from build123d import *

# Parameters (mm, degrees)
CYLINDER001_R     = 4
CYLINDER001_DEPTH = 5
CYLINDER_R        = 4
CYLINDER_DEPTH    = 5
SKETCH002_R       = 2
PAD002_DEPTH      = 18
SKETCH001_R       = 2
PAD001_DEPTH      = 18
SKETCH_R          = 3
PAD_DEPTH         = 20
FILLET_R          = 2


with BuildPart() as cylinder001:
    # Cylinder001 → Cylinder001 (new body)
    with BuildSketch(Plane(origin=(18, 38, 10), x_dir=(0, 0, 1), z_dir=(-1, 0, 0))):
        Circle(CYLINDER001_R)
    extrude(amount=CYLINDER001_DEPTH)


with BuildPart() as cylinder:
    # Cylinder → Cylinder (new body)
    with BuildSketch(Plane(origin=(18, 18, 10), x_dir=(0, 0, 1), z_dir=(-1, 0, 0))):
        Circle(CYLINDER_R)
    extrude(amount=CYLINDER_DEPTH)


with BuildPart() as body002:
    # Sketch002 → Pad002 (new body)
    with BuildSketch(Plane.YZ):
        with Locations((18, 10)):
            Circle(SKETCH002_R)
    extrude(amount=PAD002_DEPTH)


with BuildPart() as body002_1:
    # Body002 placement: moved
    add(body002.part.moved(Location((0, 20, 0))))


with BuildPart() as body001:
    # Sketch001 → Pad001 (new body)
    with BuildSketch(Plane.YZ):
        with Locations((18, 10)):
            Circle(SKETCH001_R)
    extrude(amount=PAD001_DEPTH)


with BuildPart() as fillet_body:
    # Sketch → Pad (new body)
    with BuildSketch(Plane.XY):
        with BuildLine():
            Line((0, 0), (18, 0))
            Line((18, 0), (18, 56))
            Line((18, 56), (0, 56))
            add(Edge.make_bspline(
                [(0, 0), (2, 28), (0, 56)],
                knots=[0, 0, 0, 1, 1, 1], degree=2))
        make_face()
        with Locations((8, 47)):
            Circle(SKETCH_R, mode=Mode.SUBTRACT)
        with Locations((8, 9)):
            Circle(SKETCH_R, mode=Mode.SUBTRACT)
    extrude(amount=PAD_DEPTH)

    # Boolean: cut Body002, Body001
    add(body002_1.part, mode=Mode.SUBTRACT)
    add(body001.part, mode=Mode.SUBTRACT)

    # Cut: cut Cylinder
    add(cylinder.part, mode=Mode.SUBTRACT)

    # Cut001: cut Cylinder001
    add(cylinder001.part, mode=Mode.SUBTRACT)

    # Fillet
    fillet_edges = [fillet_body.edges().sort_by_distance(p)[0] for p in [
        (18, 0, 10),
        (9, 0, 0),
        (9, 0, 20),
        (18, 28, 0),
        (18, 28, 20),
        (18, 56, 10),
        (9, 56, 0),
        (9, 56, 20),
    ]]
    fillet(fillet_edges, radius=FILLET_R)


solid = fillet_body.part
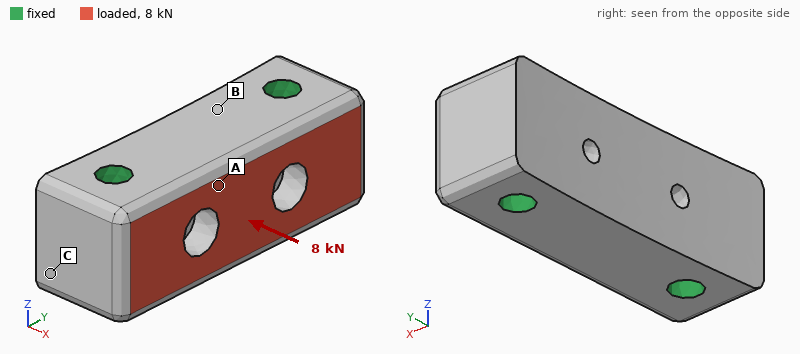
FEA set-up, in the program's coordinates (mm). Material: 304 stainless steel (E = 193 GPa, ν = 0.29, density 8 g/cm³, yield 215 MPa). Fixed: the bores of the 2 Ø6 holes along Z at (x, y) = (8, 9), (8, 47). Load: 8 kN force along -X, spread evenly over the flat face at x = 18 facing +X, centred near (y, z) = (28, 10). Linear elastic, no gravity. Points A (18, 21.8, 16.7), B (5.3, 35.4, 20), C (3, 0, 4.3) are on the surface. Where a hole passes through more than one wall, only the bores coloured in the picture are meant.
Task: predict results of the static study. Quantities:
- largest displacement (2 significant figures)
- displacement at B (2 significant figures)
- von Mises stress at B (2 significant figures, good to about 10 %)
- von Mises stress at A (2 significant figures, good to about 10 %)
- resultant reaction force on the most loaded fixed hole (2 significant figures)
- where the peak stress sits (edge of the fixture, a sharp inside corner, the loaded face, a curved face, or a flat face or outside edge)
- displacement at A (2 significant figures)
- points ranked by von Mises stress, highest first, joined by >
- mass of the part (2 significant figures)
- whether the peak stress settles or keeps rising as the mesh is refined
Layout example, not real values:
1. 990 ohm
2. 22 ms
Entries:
1. 2.2 µm
2. 1.5 µm
3. 8.9 MPa
4. 12 MPa
5. 4.0 kN
6. edge of the fixture
7. 1.9 µm
8. A > B > C
9. 140 g
10. keeps rising
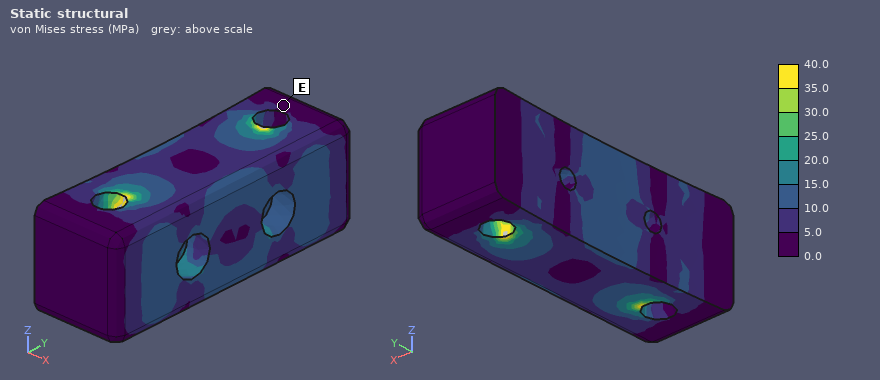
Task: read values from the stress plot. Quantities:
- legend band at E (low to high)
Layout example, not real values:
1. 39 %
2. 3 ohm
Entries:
1. 0.0 to 5.0 MPa
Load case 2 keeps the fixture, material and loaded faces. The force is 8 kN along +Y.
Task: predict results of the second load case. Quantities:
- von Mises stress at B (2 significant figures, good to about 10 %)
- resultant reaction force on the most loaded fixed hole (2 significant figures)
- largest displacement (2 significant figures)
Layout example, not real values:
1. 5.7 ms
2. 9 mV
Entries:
1. 5.5 MPa
2. 4.3 kN
3. 2.0 µm
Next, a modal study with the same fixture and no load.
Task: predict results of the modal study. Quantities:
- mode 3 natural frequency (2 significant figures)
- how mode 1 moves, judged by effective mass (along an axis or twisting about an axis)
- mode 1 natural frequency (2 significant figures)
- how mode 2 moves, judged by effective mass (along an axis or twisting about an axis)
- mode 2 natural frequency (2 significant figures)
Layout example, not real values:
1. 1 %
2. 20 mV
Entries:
1. 37 kHz
2. along X
3. 29 kHz
4. along Z
5. 31 kHz
